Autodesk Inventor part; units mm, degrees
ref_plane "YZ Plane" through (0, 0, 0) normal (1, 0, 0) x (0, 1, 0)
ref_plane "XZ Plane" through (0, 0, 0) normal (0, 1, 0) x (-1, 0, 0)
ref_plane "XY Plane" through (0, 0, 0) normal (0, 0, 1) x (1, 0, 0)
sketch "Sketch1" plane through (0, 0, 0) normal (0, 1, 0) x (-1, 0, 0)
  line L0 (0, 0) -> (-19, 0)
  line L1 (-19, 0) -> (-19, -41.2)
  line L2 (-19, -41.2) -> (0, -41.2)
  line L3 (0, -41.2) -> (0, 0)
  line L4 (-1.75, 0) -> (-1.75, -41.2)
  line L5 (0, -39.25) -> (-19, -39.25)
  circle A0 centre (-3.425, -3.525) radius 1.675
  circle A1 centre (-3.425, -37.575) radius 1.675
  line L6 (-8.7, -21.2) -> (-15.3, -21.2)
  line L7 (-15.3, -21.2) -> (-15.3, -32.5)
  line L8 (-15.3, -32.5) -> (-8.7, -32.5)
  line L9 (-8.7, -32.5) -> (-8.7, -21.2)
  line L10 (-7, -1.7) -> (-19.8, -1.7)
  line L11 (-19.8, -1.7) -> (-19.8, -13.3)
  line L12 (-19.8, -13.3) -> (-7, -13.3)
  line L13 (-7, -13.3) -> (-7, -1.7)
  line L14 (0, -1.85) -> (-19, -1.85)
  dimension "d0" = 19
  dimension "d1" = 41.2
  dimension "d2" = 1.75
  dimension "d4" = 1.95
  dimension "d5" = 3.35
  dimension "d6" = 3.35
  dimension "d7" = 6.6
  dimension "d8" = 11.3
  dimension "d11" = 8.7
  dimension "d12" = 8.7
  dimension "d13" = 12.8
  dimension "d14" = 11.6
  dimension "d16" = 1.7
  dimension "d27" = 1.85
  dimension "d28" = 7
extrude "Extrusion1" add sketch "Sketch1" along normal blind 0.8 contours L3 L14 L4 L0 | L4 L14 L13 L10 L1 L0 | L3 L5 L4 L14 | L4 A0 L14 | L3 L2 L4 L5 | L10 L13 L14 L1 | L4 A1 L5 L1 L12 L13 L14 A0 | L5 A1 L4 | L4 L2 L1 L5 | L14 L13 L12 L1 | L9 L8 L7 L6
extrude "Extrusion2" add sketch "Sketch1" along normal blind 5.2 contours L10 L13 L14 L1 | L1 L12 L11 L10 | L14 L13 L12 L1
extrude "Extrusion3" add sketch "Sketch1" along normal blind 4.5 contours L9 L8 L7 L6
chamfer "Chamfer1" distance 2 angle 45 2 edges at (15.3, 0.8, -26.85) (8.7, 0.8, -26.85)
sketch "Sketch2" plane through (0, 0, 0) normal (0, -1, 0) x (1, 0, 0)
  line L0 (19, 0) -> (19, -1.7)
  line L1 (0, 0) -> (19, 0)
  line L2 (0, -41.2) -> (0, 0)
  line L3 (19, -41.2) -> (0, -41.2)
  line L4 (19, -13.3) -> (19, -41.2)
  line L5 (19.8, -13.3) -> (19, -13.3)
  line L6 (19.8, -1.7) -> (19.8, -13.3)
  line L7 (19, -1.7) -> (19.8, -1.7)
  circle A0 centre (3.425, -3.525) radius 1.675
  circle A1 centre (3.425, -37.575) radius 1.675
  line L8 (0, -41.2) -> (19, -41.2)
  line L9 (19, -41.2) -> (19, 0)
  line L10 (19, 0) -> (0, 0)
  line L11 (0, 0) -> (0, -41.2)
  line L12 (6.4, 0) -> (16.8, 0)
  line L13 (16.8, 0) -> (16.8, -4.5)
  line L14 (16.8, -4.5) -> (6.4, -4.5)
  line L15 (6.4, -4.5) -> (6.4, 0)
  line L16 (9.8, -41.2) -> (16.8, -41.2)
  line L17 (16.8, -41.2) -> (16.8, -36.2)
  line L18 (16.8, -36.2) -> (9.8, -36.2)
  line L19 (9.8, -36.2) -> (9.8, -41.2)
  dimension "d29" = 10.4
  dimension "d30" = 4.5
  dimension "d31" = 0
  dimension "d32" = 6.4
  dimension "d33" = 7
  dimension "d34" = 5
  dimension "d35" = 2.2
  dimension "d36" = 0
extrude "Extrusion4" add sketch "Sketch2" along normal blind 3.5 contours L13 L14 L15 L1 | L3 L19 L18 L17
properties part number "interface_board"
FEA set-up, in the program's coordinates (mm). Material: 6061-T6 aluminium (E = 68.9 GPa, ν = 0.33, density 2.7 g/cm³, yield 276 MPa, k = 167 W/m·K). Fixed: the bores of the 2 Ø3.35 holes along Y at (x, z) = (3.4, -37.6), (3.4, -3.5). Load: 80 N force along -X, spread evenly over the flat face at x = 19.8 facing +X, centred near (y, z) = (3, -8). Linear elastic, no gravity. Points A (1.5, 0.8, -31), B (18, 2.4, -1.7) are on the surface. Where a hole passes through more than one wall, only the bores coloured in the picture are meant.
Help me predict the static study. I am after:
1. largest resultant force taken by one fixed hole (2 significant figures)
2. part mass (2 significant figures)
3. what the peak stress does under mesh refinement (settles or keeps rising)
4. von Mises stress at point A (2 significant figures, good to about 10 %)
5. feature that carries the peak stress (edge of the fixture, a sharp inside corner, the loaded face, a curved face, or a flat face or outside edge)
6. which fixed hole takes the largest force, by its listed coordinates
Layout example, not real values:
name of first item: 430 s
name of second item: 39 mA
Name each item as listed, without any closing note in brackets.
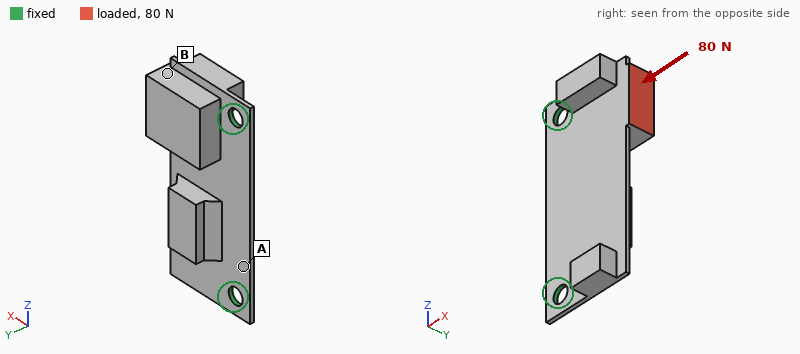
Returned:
largest resultant force taken by one fixed hole: 72 N
part mass: 5.1 g
what the peak stress does under mesh refinement: keeps rising
von Mises stress at point A: 20 MPa
feature that carries the peak stress: edge of the fixture
which fixed hole takes the largest force, by its listed coordinates: (3.4, -3.5)
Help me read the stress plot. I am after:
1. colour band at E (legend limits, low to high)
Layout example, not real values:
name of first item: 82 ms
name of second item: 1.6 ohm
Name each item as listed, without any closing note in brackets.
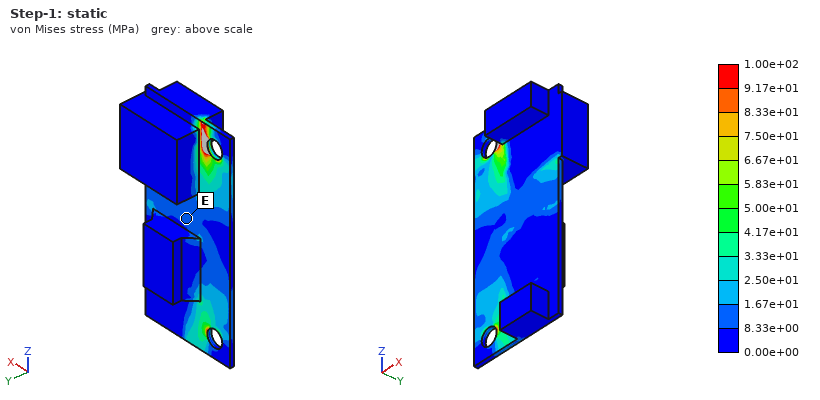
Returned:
colour band at E: 8.33e+00 to 1.67e+01 MPa
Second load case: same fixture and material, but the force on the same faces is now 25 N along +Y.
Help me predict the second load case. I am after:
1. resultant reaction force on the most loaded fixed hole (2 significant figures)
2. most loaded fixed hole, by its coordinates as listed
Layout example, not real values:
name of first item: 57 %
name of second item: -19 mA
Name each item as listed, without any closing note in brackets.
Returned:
resultant reaction force on the most loaded fixed hole: 23 N
most loaded fixed hole, by its coordinates as listed: (3.4, -3.5)
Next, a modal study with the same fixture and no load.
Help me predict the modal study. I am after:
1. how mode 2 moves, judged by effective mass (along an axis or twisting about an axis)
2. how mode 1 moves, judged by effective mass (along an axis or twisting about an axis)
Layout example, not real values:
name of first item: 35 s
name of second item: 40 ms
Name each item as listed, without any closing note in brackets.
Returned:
how mode 2 moves, judged by effective mass: twisting about X
how mode 1 moves, judged by effective mass: along Y
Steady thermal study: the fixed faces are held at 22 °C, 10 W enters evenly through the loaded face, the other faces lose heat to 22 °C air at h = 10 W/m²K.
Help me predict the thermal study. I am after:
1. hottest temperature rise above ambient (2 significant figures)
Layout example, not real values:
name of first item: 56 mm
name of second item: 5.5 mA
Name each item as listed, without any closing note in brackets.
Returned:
hottest temperature rise above ambient: 29 K
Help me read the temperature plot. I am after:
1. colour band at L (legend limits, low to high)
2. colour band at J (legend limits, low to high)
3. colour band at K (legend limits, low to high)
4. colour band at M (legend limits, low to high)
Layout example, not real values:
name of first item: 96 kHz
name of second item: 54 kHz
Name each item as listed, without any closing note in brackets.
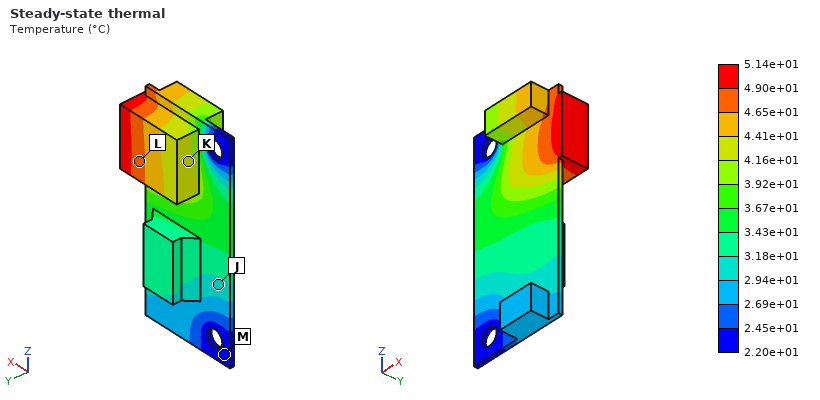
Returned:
colour band at L: 4.65e+01 to 4.90e+01 °C
colour band at J: 2.94e+01 to 3.18e+01 °C
colour band at K: 4.16e+01 to 4.41e+01 °C
colour band at M: 2.20e+01 to 2.45e+01 °C
